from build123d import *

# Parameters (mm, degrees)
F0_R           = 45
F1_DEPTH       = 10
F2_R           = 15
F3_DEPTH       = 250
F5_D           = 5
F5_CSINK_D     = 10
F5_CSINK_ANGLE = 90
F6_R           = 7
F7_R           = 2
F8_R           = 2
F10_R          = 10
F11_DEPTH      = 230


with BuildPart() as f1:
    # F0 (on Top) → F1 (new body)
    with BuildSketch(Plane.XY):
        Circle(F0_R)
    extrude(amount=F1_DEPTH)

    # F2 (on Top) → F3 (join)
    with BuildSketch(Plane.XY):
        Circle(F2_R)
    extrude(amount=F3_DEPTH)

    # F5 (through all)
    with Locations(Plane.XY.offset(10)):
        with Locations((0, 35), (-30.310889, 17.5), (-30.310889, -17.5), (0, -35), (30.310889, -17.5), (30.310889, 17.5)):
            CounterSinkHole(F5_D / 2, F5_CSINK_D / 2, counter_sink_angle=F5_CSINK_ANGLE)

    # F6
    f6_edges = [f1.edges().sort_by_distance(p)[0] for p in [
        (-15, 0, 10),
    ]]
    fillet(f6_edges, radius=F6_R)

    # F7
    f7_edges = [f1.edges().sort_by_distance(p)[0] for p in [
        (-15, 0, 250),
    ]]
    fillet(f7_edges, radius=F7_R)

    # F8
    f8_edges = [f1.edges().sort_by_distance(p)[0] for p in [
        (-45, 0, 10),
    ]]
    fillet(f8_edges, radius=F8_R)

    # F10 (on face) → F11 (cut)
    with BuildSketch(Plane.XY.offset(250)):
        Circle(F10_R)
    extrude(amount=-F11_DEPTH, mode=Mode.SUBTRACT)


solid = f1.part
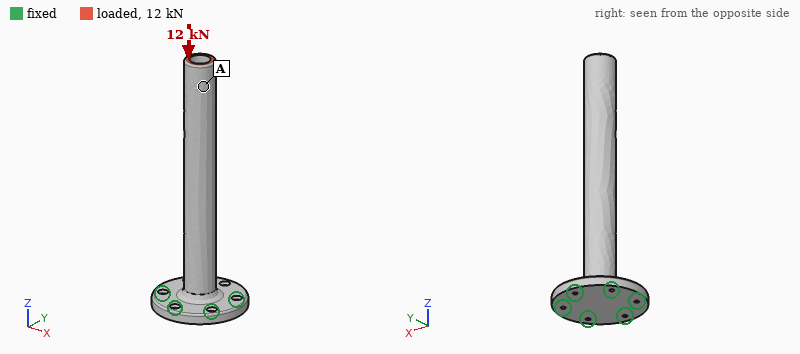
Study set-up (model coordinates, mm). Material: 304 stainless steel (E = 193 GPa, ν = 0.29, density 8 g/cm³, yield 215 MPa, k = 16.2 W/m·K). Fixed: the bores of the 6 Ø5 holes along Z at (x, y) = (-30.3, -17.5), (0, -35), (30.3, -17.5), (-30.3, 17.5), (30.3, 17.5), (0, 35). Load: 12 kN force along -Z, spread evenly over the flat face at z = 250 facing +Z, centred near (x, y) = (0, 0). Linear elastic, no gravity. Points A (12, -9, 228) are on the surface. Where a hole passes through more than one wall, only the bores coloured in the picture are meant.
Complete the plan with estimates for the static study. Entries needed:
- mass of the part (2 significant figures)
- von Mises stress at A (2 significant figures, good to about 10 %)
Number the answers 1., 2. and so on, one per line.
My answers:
1. 1.3 kg
2. 32 MPa
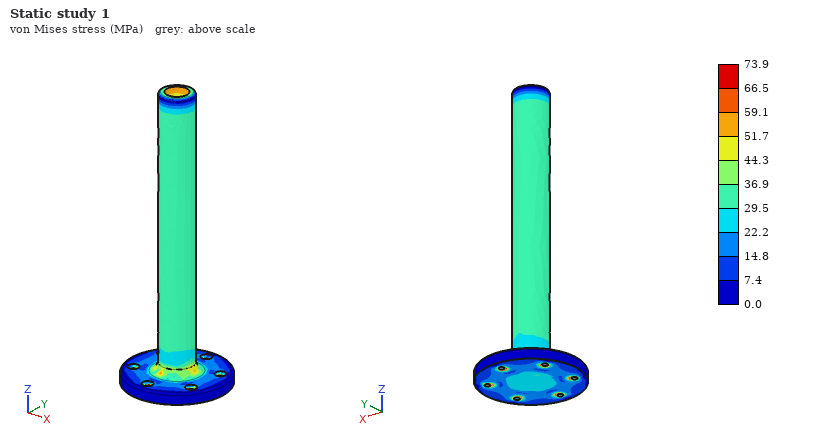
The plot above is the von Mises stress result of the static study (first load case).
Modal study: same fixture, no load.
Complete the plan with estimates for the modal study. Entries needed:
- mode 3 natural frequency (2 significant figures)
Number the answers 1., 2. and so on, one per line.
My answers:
1. 2300 Hz
